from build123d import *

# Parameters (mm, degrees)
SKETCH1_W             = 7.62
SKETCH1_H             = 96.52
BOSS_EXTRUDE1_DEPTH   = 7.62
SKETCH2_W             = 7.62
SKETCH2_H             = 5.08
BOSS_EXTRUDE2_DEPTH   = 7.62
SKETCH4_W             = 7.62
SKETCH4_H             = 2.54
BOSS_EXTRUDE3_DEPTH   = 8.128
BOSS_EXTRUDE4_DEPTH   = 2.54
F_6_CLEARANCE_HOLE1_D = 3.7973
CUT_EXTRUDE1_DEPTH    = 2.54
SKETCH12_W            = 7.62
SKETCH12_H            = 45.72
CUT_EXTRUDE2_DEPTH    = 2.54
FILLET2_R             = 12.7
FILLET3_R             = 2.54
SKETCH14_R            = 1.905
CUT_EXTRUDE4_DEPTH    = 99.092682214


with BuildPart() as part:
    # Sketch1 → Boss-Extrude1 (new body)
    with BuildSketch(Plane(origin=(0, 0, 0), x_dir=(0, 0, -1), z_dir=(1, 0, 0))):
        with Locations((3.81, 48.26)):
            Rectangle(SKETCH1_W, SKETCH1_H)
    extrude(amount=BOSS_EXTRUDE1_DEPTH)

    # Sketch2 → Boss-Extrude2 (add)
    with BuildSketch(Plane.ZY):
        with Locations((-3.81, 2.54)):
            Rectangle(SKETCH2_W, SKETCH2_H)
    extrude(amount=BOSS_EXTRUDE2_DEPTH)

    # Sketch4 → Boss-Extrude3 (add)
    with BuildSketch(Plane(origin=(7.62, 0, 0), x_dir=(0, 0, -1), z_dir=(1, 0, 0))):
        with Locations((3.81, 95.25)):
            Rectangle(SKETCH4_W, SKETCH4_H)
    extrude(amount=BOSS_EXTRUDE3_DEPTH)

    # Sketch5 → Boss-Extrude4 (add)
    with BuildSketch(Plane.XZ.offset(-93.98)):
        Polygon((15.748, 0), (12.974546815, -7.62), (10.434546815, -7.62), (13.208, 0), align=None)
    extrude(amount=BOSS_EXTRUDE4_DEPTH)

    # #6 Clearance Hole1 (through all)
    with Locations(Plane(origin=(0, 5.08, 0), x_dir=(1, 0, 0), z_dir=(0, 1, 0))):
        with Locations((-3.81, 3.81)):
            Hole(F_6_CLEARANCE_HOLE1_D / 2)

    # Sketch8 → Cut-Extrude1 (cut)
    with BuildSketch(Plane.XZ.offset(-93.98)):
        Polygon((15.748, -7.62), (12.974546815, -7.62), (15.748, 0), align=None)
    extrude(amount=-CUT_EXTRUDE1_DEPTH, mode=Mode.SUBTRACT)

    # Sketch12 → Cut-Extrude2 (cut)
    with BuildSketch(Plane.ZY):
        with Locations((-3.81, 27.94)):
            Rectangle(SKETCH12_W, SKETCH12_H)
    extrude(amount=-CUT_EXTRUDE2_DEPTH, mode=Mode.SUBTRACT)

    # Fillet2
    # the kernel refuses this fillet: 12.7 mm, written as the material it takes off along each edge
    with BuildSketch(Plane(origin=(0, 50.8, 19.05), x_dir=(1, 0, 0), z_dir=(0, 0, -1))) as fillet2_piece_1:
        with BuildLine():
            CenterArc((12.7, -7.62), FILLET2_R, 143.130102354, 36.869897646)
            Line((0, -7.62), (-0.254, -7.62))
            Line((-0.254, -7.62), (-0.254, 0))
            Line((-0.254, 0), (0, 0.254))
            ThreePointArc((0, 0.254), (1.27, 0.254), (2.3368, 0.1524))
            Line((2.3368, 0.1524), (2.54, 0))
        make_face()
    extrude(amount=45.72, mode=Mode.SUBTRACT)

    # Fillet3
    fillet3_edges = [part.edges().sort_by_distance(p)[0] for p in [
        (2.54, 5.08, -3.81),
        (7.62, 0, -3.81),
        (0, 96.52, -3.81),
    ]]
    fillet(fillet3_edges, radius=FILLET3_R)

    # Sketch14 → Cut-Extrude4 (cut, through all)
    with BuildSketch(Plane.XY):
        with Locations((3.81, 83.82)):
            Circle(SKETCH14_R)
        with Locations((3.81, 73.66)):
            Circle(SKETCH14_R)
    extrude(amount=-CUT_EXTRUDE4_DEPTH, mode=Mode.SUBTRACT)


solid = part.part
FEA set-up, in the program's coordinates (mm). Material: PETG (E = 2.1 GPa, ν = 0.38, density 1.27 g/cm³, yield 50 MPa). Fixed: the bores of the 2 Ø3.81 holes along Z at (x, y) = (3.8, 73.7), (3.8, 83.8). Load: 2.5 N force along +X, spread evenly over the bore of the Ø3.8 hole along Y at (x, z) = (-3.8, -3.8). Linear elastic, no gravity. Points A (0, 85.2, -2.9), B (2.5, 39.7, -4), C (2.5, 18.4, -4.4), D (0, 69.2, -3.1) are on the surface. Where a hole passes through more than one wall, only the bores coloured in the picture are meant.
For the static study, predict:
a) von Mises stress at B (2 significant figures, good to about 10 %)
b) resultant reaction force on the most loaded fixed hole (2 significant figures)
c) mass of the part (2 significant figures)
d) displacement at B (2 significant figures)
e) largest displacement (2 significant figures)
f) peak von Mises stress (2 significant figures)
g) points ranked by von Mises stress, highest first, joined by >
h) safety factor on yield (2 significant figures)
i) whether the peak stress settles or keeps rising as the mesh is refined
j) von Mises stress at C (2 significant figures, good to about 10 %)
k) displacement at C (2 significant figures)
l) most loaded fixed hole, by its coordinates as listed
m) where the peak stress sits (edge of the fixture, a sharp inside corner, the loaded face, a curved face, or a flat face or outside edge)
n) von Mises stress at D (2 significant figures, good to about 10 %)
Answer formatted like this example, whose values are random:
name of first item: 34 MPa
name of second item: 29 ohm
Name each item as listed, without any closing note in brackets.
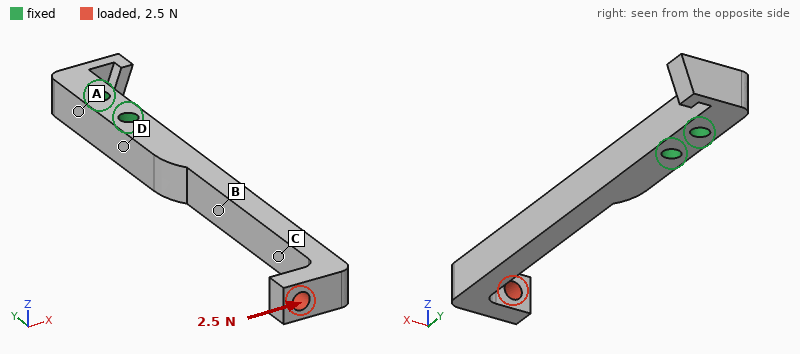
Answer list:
von Mises stress at B: 2.8 MPa
resultant reaction force on the most loaded fixed hole: 6.0 N
mass of the part: 6.2 g
displacement at B: 0.20 mm
largest displacement: 1.1 mm
peak von Mises stress: 3.7 MPa
points ranked by von Mises stress, highest first, joined by >: B > D > C > A
safety factor on yield: 14
whether the peak stress settles or keeps rising as the mesh is refined: settles
von Mises stress at C: 1.2 MPa
displacement at C: 0.59 mm
most loaded fixed hole, by its coordinates as listed: (3.8, 73.7)
where the peak stress sits: a flat face or outside edge
von Mises stress at D: 2.2 MPa
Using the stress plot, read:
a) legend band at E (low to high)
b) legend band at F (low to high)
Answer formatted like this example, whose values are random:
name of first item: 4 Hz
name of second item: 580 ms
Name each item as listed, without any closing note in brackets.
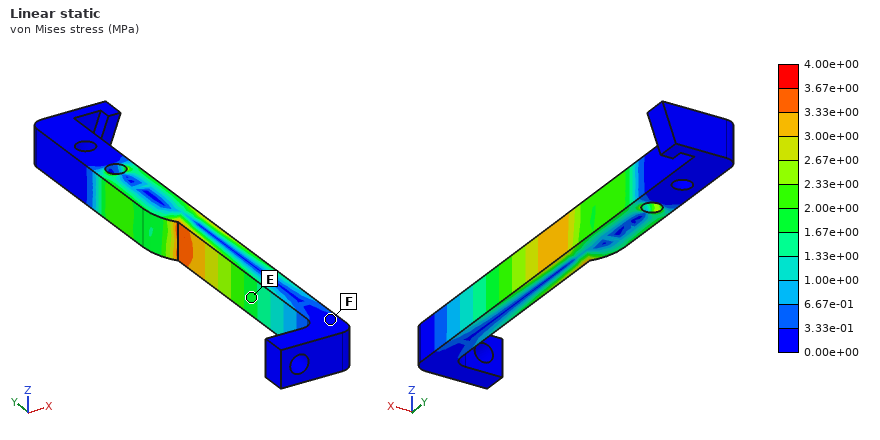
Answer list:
legend band at E: 1.67e+00 to 2.00e+00 MPa
legend band at F: 0.00e+00 to 3.33e-01 MPa
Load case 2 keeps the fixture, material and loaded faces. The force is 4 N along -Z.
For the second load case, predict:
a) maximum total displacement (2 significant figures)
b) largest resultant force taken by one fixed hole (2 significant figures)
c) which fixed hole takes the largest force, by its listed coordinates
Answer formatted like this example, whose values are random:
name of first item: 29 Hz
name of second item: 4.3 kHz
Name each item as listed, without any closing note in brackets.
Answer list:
maximum total displacement: 1.2 mm
largest resultant force taken by one fixed hole: 5.4 N
which fixed hole takes the largest force, by its listed coordinates: (3.8, 73.7)
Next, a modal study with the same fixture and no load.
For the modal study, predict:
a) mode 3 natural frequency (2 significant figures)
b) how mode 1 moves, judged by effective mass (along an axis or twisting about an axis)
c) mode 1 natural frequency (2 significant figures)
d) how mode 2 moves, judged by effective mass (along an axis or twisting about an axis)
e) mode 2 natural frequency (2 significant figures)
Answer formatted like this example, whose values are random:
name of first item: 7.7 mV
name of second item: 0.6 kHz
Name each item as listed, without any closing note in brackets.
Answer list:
mode 3 natural frequency: 1200 Hz
how mode 1 moves, judged by effective mass: along X
mode 1 natural frequency: 230 Hz
how mode 2 moves, judged by effective mass: along Z
mode 2 natural frequency: 280 Hz
